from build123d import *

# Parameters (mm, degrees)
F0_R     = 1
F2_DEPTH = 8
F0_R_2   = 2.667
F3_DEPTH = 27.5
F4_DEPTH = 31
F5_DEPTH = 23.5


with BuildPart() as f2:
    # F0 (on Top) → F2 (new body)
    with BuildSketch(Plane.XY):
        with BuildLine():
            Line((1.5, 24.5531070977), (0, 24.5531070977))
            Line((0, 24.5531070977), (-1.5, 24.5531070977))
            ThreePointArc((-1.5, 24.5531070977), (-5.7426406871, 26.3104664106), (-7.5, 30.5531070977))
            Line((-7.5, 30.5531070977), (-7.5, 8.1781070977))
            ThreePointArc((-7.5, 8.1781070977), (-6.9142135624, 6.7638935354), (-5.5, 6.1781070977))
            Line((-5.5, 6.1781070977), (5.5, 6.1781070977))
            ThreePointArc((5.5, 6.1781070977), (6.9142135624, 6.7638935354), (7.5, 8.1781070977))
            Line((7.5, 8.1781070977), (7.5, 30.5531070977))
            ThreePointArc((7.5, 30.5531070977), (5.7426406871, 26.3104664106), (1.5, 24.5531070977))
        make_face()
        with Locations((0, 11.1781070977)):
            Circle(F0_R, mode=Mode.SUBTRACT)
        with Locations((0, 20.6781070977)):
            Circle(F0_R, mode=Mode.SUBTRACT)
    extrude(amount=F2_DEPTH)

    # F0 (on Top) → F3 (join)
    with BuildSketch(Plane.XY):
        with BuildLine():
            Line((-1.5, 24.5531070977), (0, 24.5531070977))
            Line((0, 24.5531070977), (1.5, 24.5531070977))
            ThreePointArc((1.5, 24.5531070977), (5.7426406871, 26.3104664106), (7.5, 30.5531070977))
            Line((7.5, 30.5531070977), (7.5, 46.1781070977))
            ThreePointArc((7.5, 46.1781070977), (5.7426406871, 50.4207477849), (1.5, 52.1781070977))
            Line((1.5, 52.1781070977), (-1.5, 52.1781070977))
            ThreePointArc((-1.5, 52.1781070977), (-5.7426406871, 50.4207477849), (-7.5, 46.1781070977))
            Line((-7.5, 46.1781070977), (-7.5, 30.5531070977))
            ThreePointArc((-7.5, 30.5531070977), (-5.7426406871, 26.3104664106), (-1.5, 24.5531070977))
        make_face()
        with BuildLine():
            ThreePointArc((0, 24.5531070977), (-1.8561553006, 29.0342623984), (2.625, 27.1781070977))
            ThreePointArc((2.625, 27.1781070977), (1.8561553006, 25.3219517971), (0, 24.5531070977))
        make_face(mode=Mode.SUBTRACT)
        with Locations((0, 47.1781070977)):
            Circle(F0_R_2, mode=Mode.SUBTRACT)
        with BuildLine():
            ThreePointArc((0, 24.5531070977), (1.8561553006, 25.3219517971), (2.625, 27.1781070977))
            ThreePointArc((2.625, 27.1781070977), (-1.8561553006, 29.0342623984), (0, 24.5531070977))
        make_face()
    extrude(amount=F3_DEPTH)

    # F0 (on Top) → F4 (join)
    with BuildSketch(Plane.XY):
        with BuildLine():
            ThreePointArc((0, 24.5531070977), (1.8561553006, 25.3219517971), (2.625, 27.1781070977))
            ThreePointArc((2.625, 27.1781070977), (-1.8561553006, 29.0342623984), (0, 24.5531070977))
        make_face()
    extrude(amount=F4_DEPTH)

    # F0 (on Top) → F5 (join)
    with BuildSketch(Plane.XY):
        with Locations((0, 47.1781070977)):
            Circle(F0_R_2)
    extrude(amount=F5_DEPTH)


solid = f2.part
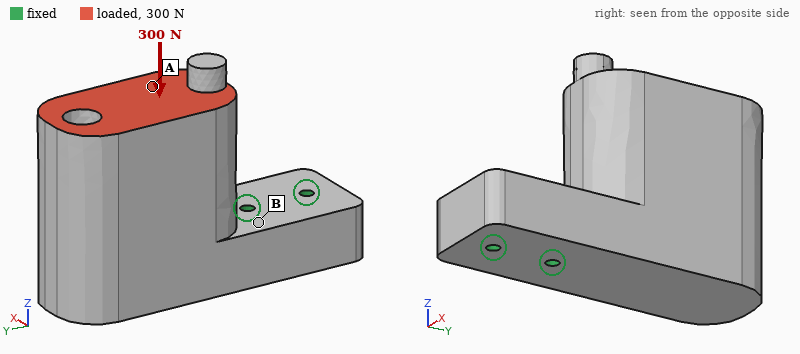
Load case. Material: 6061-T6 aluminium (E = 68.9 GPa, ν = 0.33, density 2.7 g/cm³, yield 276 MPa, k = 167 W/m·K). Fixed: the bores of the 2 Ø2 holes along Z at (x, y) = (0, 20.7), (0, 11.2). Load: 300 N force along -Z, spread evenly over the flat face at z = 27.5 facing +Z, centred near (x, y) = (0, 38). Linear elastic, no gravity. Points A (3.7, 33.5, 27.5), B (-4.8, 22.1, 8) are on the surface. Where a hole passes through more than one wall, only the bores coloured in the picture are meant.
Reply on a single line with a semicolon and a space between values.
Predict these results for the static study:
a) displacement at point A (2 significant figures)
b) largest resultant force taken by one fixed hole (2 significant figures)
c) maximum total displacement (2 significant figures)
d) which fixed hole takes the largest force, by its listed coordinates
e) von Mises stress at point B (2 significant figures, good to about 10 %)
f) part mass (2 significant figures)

26 µm; 470 N; 39 µm; (0, 20.7); 21 MPa; 35 g
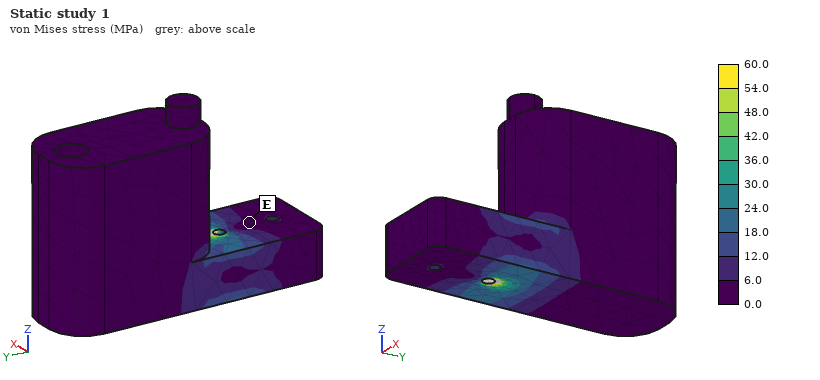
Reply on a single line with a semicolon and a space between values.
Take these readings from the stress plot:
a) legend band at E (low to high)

0.0 to 6.0 MPa
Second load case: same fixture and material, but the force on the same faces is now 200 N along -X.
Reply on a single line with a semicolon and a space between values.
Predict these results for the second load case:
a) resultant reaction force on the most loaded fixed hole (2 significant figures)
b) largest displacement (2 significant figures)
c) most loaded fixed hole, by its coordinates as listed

500 N; 37 µm; (0, 20.7)
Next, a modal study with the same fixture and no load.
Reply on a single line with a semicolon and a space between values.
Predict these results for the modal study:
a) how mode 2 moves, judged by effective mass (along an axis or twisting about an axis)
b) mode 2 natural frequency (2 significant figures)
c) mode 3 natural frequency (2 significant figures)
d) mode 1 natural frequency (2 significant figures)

along X; 3700 Hz; 7400 Hz; 3000 Hz
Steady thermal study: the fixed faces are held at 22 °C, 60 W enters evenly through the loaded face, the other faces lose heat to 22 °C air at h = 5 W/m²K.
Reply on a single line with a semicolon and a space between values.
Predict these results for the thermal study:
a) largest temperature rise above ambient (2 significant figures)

57 K
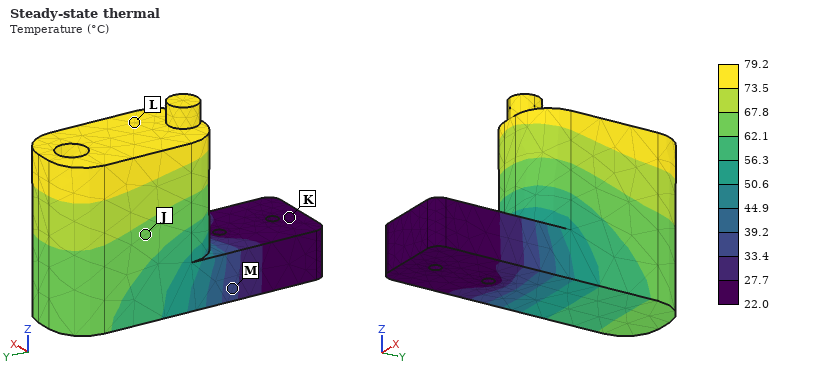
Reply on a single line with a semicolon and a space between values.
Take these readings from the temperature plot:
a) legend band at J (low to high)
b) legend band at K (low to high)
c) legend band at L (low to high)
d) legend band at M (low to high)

62.1 to 67.8 °C; 22.0 to 27.7 °C; 73.5 to 79.2 °C; 33.4 to 39.2 °C
